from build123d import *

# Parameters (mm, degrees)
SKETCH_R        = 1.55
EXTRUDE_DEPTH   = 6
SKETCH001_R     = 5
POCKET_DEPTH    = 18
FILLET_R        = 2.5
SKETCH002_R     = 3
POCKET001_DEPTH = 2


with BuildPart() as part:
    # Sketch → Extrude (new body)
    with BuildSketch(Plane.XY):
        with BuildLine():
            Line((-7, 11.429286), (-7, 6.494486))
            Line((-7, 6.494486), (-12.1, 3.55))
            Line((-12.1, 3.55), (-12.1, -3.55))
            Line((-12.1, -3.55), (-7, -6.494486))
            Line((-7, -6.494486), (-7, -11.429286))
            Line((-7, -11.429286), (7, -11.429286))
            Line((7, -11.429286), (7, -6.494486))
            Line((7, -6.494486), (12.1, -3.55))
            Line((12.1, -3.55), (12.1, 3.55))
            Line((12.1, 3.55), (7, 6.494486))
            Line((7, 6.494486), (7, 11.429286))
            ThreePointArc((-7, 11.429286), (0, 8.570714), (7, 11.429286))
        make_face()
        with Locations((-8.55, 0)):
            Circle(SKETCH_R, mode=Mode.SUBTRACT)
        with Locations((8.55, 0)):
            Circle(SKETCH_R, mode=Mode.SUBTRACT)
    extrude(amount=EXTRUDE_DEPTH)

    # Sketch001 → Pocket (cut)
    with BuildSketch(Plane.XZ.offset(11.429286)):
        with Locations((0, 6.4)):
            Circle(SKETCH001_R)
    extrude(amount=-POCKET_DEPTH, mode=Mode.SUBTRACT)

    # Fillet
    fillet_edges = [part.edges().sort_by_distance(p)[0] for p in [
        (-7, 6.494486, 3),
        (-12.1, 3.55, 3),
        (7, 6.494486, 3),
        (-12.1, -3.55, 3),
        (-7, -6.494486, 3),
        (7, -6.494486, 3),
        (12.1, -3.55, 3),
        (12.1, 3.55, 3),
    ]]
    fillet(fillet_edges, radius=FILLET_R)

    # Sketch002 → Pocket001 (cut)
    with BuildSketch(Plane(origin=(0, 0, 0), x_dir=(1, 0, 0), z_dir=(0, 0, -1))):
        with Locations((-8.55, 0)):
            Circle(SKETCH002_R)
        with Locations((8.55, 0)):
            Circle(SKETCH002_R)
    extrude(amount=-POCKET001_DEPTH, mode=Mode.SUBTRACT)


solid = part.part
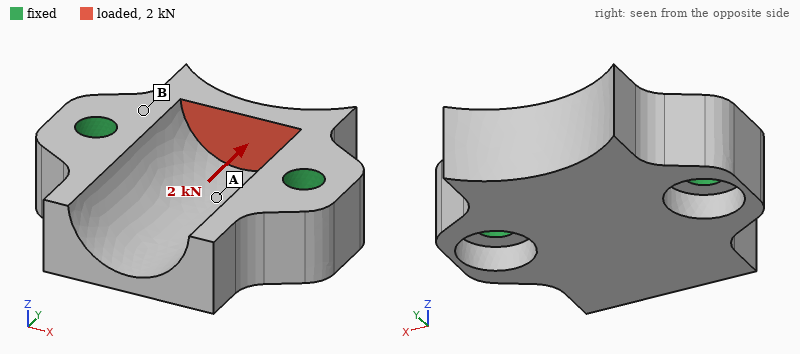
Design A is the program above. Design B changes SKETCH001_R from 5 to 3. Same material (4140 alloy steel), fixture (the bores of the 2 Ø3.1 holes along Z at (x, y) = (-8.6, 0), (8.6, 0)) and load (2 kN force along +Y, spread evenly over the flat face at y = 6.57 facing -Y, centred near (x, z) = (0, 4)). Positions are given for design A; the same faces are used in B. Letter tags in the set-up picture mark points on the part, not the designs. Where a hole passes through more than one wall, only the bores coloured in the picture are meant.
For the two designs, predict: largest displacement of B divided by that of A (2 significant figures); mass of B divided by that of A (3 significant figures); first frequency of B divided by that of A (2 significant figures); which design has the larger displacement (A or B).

0.80
1.27
0.90
A
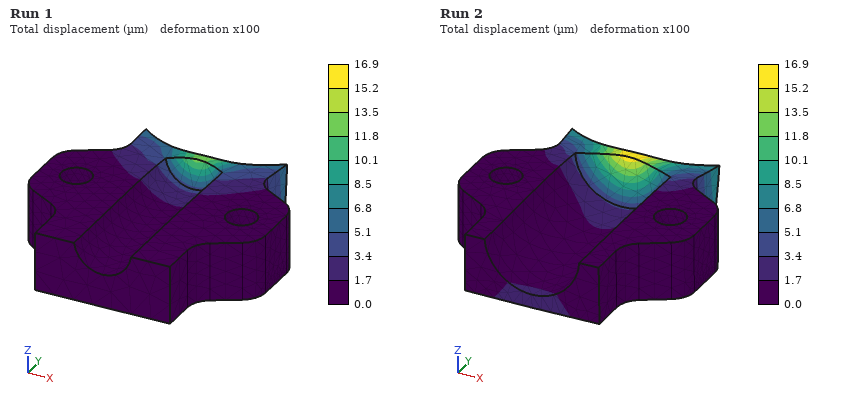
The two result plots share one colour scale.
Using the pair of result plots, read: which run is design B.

Run 1
